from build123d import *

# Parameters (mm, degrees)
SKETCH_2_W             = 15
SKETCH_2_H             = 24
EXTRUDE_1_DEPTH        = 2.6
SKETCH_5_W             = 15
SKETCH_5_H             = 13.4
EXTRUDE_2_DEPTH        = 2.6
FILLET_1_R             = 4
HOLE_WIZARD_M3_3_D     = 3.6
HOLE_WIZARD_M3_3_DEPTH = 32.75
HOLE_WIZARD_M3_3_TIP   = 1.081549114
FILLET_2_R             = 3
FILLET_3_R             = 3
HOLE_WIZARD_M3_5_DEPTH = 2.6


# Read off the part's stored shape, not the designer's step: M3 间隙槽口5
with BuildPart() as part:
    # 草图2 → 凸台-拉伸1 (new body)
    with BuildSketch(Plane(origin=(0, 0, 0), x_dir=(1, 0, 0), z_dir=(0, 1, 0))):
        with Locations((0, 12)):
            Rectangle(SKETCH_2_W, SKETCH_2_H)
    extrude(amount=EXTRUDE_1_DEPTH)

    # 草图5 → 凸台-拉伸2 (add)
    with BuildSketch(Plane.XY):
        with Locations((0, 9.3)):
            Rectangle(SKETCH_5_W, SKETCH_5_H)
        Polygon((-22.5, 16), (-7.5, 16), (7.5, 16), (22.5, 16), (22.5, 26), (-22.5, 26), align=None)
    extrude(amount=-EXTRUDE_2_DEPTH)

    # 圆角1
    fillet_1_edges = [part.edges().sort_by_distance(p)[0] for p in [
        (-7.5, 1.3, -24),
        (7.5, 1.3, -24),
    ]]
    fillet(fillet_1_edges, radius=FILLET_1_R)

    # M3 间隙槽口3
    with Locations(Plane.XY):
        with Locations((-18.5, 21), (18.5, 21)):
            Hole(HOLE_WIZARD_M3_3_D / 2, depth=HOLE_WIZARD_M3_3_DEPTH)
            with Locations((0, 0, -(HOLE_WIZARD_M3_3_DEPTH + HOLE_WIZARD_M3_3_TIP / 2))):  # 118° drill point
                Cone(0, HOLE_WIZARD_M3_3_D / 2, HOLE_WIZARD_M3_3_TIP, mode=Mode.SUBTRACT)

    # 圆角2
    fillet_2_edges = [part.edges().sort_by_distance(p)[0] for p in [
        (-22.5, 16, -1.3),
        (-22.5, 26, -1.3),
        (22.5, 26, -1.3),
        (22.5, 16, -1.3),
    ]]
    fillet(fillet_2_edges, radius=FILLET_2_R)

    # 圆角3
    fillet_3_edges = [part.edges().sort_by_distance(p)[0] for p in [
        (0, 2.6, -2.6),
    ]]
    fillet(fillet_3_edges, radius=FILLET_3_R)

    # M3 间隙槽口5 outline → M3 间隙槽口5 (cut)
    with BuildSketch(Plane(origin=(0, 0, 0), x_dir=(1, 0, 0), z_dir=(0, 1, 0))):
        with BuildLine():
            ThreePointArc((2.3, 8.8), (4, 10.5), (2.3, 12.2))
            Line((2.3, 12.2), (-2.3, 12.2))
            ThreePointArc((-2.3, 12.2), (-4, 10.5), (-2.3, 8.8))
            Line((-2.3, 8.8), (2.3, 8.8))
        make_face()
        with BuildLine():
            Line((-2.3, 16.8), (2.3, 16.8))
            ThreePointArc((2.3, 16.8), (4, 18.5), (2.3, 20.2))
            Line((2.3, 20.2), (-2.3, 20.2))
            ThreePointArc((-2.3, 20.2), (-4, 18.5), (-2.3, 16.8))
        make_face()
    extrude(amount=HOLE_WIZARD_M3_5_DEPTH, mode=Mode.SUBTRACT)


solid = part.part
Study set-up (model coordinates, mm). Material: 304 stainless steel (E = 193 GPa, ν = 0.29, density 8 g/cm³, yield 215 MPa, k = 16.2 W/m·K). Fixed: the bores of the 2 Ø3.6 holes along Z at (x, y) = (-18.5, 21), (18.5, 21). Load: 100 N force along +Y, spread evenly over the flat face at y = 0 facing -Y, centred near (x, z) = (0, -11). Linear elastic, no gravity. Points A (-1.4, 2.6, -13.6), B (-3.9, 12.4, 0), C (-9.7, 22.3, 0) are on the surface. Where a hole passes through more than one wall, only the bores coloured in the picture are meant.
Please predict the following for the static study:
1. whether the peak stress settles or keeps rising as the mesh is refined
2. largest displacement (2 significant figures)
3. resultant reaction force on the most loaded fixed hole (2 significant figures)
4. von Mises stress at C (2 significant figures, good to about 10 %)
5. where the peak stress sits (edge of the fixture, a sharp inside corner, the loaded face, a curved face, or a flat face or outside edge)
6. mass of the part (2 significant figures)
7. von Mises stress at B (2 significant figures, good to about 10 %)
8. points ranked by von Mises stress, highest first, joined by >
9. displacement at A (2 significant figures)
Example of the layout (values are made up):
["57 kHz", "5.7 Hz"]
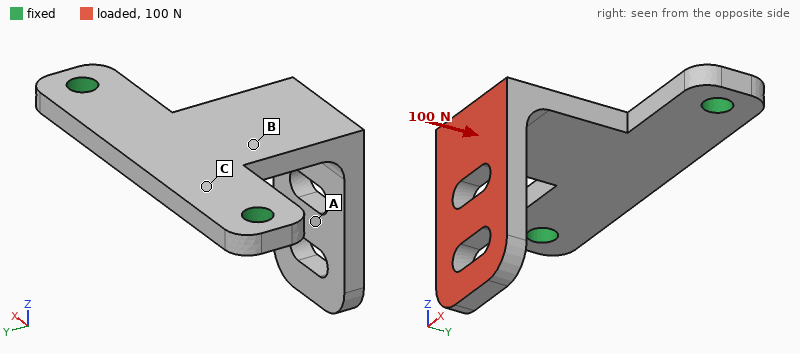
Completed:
["keeps rising", "0.17 mm", "52 N", "32 MPa", "a sharp inside corner", "20 g", "57 MPa", "B > C > A", "0.093 mm"]
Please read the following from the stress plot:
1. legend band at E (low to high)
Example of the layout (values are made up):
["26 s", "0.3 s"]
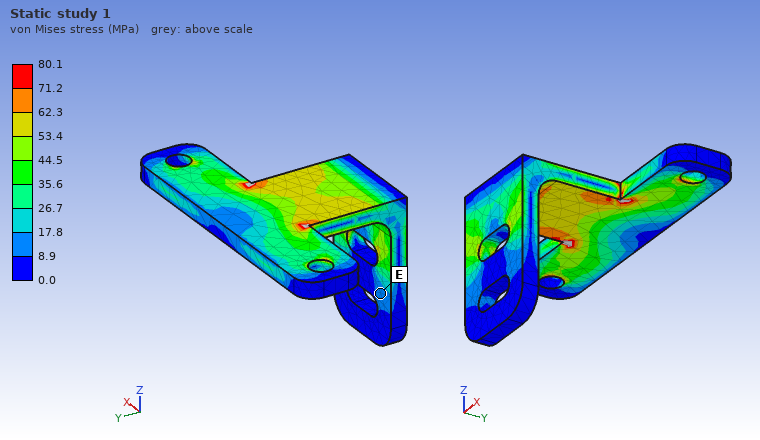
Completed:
["8.9 to 17.8 MPa"]
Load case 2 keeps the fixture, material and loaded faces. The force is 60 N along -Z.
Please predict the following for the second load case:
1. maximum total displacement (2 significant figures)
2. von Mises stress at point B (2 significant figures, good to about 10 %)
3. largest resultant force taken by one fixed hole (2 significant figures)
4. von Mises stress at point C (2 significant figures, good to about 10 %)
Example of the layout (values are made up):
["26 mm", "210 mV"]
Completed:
["0.13 mm", "48 MPa", "30 N", "44 MPa"]
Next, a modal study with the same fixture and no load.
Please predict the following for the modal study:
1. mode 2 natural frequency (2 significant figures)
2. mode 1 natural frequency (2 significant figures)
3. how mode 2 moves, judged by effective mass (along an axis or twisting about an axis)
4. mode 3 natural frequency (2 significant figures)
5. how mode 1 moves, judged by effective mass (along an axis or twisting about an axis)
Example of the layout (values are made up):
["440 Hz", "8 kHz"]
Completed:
["3100 Hz", "1400 Hz", "along X", "3900 Hz", "along Z"]
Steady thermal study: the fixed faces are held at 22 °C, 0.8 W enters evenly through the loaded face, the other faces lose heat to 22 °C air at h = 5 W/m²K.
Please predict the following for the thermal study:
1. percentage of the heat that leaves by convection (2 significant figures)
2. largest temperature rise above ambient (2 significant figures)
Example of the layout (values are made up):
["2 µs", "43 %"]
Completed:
["21 %", "41 K"]
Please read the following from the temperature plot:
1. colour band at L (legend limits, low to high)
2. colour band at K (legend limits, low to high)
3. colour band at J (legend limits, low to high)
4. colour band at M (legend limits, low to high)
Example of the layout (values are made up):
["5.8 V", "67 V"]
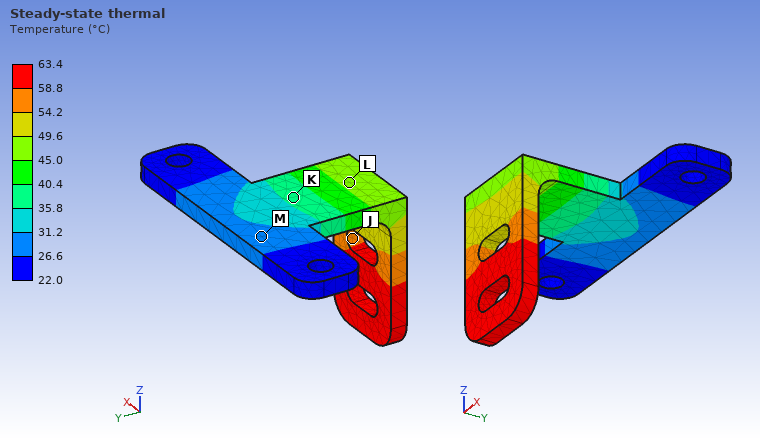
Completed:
["45.0 to 49.6 °C", "35.8 to 40.4 °C", "54.2 to 58.8 °C", "26.6 to 31.2 °C"]
